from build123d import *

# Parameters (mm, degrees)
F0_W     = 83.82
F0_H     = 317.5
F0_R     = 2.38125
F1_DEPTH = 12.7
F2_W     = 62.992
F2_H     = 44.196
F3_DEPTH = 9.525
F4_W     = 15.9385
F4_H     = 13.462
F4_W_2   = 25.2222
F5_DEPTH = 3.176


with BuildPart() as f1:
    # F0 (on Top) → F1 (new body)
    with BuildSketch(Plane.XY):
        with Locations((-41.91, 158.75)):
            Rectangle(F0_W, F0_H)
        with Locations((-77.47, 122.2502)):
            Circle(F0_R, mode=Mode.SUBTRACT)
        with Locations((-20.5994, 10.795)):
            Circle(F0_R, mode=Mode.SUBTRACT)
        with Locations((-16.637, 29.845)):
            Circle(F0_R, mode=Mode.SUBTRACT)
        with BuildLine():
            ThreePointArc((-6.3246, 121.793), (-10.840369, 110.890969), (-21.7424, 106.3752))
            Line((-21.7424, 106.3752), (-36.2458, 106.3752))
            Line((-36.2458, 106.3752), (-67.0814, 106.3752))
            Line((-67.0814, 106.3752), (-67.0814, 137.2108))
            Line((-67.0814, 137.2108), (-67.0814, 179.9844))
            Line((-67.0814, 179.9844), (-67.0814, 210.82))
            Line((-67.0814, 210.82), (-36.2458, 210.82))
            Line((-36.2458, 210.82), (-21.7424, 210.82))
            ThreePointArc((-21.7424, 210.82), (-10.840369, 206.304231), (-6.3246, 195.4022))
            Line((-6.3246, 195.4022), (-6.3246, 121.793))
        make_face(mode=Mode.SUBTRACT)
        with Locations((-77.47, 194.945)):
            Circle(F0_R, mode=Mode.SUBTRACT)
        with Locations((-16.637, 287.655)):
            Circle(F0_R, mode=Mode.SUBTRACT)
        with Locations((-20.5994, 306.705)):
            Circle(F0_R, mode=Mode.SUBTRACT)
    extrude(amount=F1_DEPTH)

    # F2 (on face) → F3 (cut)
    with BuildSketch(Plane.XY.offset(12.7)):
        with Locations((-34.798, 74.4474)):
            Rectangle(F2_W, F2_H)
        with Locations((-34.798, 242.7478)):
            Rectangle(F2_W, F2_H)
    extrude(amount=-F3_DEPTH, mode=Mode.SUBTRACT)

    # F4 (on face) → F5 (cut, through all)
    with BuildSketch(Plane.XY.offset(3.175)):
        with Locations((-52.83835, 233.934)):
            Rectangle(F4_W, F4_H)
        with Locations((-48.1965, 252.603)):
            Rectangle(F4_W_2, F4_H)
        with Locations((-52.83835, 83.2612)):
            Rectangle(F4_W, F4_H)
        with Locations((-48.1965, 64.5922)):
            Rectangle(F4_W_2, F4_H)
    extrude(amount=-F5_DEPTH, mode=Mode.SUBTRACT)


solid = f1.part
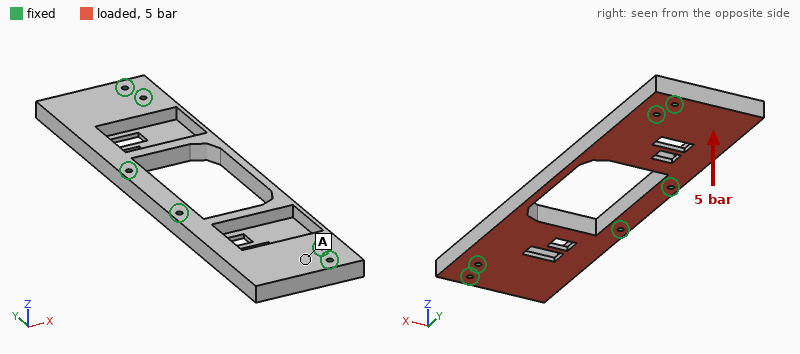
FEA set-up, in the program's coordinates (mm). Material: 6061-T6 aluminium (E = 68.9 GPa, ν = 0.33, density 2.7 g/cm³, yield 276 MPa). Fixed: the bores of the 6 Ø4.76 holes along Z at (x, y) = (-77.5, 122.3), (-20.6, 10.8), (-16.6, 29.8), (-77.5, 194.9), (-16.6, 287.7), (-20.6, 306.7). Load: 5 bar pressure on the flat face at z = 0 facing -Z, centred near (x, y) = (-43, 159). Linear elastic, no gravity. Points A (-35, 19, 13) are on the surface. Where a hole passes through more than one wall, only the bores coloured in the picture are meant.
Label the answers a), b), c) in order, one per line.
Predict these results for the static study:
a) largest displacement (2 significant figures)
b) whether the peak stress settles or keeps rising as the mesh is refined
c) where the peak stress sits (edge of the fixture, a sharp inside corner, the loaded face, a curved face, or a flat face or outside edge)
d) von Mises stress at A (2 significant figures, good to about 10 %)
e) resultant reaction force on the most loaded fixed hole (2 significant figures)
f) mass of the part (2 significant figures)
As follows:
a) 0.32 mm
b) keeps rising
c) edge of the fixture
d) 16 MPa
e) 2.9 kN
f) 540 g
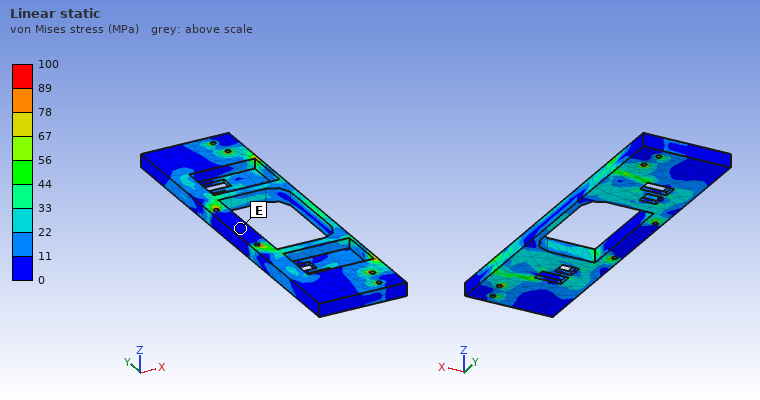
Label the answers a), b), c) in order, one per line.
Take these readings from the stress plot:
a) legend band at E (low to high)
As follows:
a) 0 to 11 MPa
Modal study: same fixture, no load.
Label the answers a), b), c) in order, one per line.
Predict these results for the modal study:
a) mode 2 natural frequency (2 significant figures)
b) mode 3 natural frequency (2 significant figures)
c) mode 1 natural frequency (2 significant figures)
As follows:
a) 2400 Hz
b) 2500 Hz
c) 1500 Hz
